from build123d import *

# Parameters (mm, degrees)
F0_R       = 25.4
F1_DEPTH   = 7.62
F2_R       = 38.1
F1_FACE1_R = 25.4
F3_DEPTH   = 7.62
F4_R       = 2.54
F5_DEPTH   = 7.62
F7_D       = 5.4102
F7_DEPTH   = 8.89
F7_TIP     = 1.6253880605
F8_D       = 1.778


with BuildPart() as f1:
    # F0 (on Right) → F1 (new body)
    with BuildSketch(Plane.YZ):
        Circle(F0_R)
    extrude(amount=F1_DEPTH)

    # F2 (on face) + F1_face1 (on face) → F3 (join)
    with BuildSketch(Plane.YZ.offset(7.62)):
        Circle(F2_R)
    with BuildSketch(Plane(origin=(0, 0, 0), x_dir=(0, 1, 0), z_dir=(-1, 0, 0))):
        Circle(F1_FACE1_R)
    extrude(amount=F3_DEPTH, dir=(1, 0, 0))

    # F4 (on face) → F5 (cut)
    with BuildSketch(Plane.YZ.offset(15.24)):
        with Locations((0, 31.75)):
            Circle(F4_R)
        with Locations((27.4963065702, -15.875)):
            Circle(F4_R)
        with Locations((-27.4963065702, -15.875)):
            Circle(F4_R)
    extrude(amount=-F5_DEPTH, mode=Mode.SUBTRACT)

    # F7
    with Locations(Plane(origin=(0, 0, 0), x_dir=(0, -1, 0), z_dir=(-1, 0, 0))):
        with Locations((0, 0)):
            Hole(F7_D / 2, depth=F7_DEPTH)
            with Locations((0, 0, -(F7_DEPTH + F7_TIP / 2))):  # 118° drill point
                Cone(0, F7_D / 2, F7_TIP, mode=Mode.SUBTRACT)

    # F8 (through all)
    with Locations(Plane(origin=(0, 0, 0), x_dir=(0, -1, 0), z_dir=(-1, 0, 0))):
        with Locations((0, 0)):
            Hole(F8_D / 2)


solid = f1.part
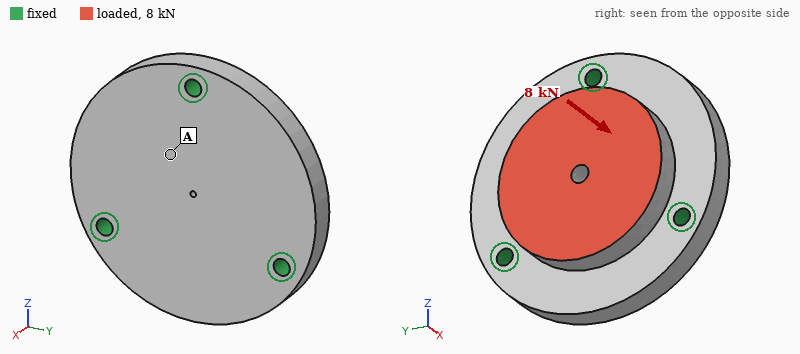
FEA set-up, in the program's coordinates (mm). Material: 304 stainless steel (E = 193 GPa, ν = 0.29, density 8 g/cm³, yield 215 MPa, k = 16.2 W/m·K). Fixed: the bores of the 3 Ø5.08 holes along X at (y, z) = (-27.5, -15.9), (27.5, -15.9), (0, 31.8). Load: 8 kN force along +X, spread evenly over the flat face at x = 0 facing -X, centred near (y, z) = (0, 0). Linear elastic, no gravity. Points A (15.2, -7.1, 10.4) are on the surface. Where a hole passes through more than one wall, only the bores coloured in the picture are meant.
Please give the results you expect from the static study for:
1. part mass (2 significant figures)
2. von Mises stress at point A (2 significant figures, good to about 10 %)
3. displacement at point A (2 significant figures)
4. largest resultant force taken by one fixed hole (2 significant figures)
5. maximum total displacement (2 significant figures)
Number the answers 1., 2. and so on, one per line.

1. 400 g
2. 13 MPa
3. 6.2 µm
4. 2.9 kN
5. 6.8 µm
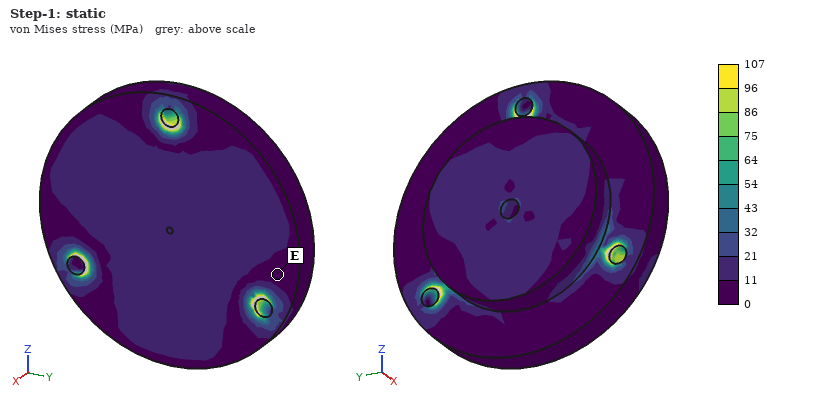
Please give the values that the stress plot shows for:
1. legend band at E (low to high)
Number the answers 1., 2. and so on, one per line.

1. 0 to 11 MPa
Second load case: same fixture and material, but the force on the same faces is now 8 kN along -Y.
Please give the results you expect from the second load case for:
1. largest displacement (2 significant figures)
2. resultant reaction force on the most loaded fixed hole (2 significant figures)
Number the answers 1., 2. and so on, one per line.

1. 6.7 µm
2. 3.4 kN
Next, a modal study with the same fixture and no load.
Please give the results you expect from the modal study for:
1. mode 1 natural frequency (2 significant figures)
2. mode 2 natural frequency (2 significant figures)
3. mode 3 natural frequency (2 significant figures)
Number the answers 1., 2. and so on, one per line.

1. 10000 Hz
2. 10000 Hz
3. 10 kHz
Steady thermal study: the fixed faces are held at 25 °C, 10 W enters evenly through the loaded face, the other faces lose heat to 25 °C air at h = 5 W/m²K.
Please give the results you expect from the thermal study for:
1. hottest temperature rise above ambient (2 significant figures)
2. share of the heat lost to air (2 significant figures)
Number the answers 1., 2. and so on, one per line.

1. 16 K
2. 4.6 %
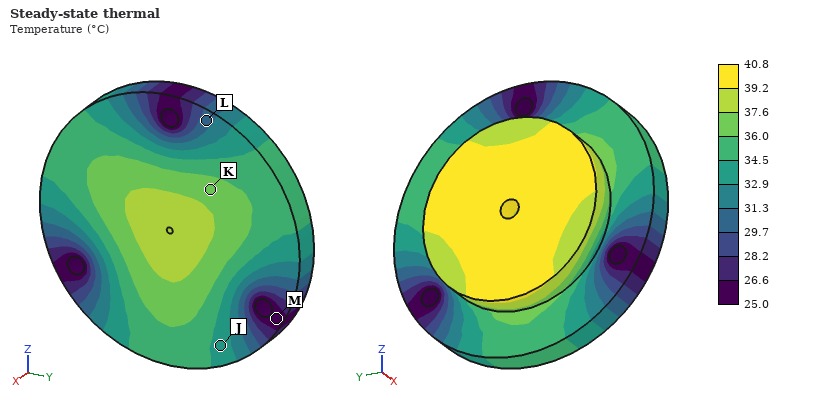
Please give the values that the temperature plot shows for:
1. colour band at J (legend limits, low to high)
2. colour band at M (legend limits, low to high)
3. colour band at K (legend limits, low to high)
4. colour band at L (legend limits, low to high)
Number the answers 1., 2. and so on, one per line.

1. 32.9 to 34.5 °C
2. 25.0 to 26.6 °C
3. 36.0 to 37.6 °C
4. 29.7 to 31.3 °C
